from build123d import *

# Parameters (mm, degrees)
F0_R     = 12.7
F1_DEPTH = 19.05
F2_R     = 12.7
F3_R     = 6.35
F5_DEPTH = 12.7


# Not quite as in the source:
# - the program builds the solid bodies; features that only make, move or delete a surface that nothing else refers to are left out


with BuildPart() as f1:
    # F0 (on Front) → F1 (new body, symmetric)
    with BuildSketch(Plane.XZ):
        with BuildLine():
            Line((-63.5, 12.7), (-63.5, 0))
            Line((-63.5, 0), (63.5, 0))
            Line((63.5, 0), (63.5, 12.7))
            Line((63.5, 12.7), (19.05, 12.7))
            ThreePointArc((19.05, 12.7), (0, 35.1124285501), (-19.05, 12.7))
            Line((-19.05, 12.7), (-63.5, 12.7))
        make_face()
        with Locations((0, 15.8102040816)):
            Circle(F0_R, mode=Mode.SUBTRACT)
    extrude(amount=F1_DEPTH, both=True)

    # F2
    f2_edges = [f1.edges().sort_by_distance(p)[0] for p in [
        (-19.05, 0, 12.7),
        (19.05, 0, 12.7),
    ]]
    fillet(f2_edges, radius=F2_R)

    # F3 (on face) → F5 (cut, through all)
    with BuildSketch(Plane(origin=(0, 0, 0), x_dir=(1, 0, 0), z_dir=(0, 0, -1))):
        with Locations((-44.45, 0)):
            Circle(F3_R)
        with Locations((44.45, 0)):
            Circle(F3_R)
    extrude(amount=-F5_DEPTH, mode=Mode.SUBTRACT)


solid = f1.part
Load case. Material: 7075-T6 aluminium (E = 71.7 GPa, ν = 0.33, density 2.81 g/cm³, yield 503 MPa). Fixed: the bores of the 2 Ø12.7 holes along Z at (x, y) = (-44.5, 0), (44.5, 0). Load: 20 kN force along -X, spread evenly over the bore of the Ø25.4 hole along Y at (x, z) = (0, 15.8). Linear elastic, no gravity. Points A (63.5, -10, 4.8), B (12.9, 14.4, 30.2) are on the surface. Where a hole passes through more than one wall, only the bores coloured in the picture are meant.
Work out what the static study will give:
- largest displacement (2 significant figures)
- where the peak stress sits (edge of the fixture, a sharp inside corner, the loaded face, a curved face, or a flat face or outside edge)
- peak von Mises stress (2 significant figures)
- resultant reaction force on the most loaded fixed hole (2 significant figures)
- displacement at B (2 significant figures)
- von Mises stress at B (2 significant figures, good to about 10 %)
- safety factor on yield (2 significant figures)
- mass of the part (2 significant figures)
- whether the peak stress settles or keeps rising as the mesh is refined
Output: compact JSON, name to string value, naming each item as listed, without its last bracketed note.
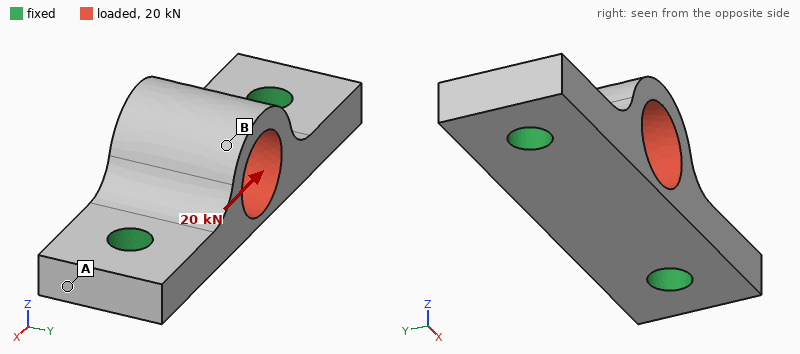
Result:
{"largest displacement": "38 µm", "where the peak stress sits": "a curved face", "peak von Mises stress": "67 MPa", "resultant reaction force on the most loaded fixed hole": "10 kN", "displacement at B": "36 µm", "von Mises stress at B": "38 MPa", "safety factor on yield": "7.6", "mass of the part": "190 g", "whether the peak stress settles or keeps rising as the mesh is refined": "settles"}
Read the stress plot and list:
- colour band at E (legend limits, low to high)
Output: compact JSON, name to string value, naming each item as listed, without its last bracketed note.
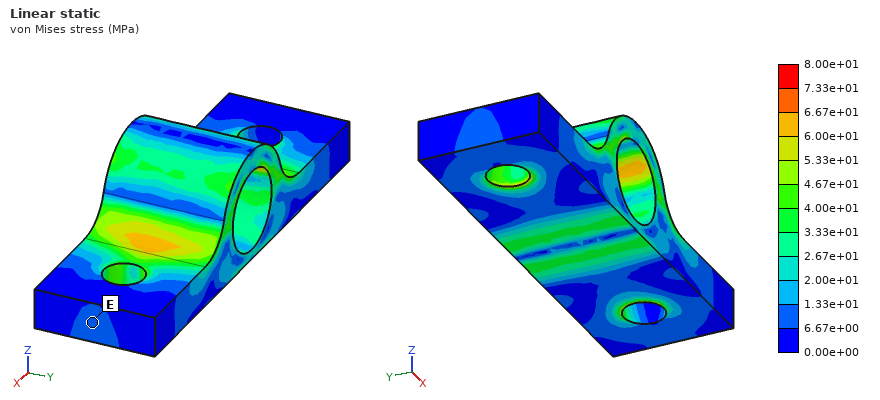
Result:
{"colour band at E": "6.67e+00 to 1.33e+01 MPa"}
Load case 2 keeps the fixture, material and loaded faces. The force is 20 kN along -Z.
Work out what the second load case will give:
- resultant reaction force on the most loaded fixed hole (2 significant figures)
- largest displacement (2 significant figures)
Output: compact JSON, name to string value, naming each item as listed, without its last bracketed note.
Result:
{"resultant reaction force on the most loaded fixed hole": "10 kN", "largest displacement": "0.11 mm"}
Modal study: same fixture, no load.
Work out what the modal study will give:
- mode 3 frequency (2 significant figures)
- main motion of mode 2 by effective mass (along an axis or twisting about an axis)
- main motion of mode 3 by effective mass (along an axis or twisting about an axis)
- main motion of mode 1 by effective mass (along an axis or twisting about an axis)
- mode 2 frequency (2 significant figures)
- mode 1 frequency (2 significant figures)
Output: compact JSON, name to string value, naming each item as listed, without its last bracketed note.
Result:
{"mode 3 frequency": "11 kHz", "main motion of mode 2 by effective mass": "along Z", "main motion of mode 3 by effective mass": "along Y", "main motion of mode 1 by effective mass": "along Y", "mode 2 frequency": "8700 Hz", "mode 1 frequency": "6900 Hz"}
